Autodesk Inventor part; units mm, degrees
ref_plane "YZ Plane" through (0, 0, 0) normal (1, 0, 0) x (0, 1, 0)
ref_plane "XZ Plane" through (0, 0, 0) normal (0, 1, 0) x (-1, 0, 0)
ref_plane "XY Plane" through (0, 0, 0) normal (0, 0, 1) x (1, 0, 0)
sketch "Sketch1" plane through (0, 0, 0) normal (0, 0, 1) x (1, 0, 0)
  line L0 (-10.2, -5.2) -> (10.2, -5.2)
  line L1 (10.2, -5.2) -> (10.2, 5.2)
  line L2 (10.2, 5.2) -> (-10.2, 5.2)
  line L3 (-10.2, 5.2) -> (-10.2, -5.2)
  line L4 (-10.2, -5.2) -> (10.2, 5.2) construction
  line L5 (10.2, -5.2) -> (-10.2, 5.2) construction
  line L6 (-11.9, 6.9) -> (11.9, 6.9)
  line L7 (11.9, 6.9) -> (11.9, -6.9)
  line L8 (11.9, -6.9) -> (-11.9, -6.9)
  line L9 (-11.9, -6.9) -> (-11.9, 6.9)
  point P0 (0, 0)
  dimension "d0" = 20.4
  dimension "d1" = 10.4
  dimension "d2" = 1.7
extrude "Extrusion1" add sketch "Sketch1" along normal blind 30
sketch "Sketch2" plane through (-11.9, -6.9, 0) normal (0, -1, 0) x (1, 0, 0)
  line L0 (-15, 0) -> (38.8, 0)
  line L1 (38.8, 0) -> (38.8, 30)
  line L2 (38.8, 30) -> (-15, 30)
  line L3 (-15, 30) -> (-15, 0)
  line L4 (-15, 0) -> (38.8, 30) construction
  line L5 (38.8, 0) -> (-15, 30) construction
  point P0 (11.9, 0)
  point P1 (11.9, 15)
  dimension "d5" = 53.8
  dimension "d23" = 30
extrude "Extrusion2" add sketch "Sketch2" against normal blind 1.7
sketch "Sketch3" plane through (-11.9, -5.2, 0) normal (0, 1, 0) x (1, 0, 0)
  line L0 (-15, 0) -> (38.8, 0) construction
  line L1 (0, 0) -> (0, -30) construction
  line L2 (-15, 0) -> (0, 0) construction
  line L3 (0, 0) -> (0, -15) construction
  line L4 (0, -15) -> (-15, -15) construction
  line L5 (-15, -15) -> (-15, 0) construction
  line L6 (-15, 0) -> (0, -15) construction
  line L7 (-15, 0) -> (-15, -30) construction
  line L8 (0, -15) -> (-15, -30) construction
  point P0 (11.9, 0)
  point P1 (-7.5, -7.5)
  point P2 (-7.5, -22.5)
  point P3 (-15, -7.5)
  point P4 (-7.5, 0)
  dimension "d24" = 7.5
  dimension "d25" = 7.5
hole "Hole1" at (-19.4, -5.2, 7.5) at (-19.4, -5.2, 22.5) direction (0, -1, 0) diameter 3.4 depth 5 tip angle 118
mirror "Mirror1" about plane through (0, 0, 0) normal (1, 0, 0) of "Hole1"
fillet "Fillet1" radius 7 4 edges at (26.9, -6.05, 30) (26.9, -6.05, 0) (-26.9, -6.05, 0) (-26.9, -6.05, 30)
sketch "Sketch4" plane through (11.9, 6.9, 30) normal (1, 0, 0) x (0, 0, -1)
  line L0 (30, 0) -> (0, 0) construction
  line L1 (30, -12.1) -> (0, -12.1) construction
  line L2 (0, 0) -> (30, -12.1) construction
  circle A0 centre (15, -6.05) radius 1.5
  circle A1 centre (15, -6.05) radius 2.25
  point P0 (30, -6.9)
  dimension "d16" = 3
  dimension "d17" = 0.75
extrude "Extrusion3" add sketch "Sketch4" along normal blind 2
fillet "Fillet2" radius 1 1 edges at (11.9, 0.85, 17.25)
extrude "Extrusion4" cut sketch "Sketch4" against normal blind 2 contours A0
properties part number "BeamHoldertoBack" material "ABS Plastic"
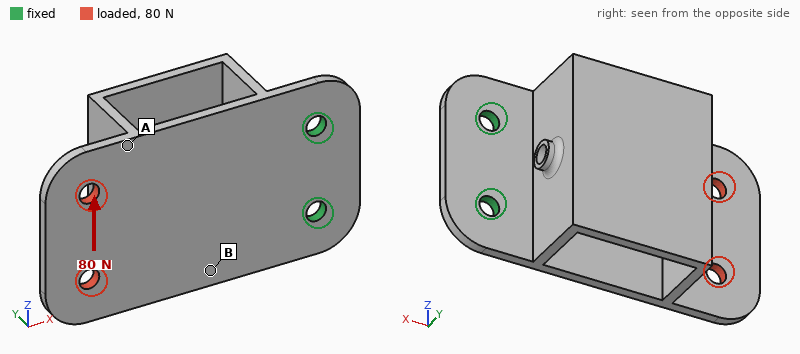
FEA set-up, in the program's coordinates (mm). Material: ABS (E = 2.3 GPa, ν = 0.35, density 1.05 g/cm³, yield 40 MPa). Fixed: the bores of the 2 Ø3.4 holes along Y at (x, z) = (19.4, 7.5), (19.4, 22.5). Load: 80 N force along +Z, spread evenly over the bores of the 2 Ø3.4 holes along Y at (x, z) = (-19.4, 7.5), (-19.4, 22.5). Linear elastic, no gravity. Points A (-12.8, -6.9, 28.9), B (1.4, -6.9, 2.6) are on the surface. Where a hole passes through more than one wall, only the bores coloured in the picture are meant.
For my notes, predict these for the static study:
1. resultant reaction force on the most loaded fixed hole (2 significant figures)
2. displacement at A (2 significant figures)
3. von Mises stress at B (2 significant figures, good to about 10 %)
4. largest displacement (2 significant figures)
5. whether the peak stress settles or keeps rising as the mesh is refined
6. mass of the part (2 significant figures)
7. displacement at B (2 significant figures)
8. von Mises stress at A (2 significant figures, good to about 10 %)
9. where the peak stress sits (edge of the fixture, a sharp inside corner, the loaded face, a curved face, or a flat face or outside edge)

180 N
0.29 mm
5.5 MPa
0.41 mm
keeps rising
5.1 g
0.15 mm
2.1 MPa
edge of the fixture
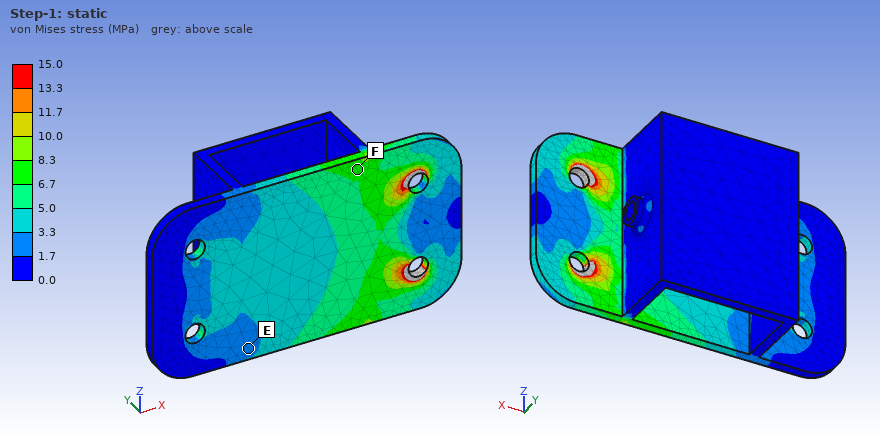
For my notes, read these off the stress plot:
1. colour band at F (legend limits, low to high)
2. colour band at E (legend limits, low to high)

6.7 to 8.3 MPa
1.7 to 3.3 MPa
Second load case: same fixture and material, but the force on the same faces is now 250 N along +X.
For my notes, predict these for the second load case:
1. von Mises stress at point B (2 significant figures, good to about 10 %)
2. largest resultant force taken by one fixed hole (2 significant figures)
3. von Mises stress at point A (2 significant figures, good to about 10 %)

4.9 MPa
130 N
4.2 MPa
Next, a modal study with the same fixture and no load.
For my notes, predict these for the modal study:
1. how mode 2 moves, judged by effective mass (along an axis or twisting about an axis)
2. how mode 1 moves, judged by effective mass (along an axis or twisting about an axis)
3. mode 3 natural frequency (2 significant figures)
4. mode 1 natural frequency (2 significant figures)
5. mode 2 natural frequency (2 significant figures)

along Z
along Y
1600 Hz
190 Hz
960 Hz
